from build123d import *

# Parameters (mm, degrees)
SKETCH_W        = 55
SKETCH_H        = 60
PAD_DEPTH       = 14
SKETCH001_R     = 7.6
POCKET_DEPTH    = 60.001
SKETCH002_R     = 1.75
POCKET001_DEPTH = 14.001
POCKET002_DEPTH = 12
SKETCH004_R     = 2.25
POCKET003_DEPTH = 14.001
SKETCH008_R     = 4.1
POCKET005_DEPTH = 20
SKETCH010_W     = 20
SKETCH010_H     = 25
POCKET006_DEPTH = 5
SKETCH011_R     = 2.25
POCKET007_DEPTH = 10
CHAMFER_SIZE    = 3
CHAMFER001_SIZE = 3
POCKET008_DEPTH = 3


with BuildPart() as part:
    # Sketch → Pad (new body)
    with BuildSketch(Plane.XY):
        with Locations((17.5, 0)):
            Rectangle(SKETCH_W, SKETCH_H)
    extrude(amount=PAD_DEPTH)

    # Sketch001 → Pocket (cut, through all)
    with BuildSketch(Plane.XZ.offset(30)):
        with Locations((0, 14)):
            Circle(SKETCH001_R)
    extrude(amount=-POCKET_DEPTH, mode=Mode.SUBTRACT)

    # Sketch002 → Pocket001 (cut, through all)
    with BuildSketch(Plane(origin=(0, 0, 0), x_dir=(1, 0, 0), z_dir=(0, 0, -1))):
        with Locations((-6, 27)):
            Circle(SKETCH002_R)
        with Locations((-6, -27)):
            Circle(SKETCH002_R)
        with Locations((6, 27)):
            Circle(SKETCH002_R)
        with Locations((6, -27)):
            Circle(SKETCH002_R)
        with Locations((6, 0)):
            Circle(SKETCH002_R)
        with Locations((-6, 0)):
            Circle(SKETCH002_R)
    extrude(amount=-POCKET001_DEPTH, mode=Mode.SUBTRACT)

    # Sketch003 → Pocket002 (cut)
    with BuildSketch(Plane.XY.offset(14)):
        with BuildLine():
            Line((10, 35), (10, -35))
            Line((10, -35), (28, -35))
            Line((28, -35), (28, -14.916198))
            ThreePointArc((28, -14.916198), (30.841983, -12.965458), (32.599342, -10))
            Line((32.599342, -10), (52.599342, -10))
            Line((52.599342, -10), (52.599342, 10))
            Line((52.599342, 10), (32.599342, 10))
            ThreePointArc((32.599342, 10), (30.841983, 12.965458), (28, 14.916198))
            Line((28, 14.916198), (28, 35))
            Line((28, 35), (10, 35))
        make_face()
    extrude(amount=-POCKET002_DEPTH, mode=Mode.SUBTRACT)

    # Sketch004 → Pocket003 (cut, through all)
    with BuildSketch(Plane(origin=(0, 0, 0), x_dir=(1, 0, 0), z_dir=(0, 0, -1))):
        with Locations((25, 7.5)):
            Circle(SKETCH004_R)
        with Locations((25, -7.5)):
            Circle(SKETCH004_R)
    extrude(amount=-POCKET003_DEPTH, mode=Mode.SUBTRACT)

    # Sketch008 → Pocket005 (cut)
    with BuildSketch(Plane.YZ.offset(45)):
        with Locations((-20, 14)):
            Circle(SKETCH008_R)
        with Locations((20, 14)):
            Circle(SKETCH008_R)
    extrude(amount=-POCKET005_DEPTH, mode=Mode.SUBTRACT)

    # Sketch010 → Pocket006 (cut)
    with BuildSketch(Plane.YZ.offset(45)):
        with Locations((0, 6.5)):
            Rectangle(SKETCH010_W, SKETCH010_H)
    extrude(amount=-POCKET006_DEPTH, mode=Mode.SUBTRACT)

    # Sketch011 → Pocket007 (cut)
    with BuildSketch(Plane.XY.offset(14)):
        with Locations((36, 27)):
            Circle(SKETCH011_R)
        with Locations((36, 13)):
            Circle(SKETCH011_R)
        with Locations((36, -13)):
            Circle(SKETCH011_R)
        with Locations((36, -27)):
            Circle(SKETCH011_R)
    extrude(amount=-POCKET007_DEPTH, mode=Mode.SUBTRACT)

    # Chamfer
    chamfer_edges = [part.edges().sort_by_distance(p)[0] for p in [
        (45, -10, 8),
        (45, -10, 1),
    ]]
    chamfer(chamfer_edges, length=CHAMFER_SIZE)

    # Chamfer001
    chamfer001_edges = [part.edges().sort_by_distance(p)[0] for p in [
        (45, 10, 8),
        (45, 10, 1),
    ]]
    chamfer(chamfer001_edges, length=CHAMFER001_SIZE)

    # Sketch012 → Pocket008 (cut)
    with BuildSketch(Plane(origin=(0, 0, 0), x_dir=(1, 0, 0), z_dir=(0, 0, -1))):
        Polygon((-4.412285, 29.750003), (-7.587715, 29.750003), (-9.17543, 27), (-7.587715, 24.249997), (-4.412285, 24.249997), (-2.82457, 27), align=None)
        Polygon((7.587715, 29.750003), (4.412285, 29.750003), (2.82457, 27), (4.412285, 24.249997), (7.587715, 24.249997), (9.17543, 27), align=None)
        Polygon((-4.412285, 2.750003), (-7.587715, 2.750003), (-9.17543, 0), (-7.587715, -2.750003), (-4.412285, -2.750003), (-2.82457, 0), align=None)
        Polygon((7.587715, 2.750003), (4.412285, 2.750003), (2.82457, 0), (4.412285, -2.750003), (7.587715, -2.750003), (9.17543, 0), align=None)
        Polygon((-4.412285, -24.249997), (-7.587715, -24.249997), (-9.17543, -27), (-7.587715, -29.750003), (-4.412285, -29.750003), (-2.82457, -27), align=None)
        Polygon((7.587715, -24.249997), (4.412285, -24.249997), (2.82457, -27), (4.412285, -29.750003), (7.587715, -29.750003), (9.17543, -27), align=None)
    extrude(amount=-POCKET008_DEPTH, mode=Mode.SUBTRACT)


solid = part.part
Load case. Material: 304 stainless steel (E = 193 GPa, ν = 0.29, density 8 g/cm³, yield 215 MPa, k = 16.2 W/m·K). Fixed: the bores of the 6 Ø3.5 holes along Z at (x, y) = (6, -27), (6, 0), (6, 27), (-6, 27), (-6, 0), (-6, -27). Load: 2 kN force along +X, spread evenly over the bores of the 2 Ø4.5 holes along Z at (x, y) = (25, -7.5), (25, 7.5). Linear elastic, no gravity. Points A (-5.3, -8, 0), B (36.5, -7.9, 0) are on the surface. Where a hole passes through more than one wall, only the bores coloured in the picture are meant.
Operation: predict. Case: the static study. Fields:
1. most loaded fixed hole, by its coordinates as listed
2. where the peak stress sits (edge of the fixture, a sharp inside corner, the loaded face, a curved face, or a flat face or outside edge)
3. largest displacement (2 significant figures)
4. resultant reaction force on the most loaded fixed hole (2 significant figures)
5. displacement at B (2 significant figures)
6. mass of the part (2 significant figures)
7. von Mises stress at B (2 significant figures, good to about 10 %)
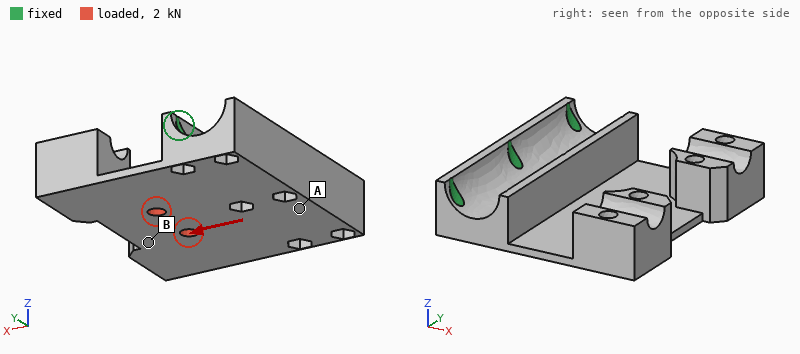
(6, 0)
the loaded face
9.7 µm
670 N
8.1 µm
160 g
11 MPa
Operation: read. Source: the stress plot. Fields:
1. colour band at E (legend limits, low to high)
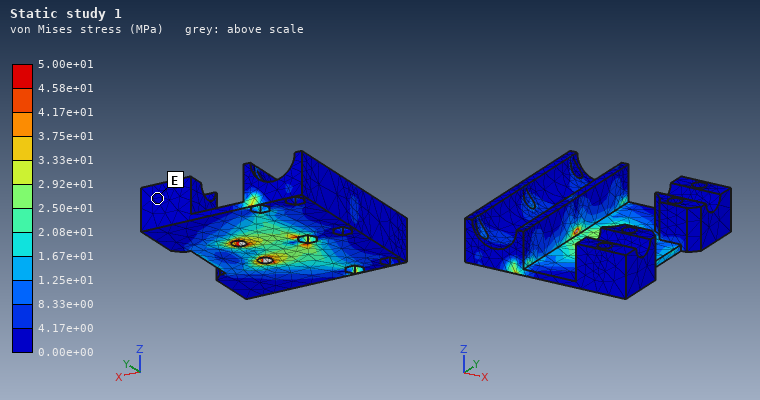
0.00e+00 to 4.17e+00 MPa
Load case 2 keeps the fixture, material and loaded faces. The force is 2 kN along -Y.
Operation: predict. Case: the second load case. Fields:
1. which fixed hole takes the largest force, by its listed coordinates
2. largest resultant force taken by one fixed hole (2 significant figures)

(6, 0)
900 N
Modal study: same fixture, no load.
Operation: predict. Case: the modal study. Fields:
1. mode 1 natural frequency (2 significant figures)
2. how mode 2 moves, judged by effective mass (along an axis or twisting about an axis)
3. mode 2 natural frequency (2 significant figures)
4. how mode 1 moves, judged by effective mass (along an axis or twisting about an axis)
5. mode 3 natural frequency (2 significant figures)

610 Hz
twisting about X
990 Hz
along Z
2400 Hz
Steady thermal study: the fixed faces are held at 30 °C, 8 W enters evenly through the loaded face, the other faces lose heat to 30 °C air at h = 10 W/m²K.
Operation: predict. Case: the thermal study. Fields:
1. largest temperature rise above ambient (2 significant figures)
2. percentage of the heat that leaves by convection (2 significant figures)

82 K
34 %
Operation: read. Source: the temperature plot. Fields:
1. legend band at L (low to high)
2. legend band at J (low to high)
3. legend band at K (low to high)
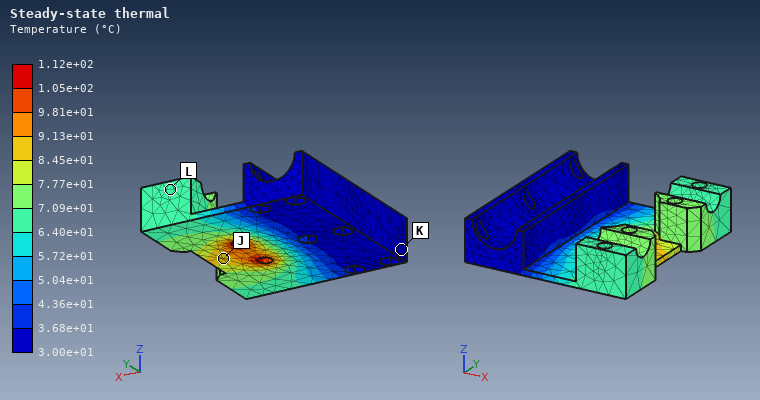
6.40e+01 to 7.09e+01 °C
8.45e+01 to 9.13e+01 °C
3.00e+01 to 3.68e+01 °C
